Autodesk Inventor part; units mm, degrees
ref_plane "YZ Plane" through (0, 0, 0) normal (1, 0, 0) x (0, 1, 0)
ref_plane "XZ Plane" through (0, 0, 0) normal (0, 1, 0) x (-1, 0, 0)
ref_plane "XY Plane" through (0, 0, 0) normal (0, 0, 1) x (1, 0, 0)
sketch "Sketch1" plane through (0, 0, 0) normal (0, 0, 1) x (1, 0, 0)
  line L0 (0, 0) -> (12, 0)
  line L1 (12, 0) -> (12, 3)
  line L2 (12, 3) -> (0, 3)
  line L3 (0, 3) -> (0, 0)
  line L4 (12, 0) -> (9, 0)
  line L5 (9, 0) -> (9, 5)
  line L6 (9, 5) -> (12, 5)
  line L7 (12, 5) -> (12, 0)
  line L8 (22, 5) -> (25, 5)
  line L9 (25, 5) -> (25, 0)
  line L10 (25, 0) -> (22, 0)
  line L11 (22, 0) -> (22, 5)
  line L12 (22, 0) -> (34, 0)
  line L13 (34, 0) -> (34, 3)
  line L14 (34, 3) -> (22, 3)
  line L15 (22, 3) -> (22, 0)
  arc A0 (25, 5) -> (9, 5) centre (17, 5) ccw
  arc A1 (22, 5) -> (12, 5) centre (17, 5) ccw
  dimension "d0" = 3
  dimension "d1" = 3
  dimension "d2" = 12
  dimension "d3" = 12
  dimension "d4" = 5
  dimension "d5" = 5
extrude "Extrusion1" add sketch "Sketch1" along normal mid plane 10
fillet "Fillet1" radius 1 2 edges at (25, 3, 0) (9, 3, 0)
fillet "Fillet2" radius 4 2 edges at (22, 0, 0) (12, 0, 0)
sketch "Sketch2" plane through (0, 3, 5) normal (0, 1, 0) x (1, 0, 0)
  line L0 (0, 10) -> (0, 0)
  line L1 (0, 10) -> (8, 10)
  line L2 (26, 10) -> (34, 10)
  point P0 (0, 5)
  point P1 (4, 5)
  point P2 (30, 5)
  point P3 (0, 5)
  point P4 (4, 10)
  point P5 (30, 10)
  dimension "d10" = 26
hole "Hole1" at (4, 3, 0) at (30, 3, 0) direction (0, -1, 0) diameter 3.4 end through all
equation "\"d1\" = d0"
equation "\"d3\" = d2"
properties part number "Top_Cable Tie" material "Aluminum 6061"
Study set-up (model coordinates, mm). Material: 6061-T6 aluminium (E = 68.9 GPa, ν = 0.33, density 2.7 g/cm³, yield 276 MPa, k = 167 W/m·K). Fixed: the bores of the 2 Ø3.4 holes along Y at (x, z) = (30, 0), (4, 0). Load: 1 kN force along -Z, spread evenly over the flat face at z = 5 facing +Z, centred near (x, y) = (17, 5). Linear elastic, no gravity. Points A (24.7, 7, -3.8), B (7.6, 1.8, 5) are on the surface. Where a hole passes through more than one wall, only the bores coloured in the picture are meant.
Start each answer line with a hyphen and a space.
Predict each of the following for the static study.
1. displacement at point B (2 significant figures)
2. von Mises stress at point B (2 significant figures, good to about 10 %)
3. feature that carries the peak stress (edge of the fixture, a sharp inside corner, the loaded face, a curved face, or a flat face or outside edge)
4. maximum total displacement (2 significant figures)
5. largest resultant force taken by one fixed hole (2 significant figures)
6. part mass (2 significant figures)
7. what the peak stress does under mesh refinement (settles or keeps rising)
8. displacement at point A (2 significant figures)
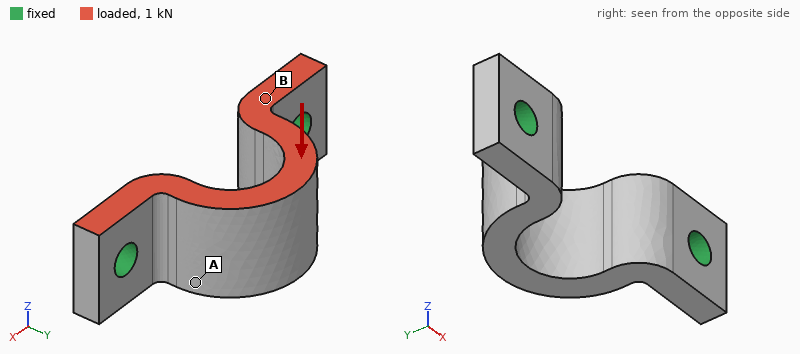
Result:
- 13 µm
- 88 MPa
- edge of the fixture
- 58 µm
- 500 N
- 3.6 g
- keeps rising
- 31 µm
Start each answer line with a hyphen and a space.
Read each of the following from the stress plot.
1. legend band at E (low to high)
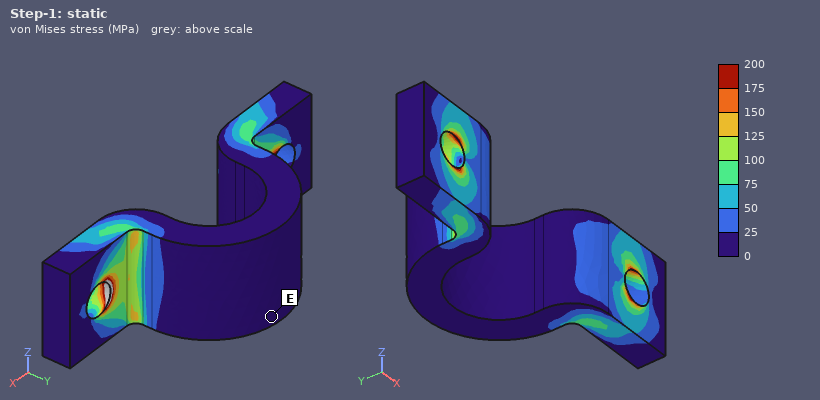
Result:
- 0 to 25 MPa
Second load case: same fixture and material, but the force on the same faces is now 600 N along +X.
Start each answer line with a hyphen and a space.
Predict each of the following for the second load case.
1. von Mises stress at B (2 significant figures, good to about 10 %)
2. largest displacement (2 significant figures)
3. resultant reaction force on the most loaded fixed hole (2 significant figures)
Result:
- 17 MPa
- 14 µm
- 320 N
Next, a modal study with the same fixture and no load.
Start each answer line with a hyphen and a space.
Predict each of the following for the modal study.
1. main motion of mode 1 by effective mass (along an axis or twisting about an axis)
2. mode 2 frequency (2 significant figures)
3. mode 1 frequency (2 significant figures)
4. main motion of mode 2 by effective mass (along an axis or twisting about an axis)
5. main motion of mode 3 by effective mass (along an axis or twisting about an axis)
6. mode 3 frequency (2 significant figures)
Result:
- along Z
- 26 kHz
- 13 kHz
- along X
- along Y
- 30 kHz
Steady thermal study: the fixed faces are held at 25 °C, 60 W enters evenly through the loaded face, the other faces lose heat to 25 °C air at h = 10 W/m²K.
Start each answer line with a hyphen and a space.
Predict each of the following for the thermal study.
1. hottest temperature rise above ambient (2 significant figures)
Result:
- 53 K
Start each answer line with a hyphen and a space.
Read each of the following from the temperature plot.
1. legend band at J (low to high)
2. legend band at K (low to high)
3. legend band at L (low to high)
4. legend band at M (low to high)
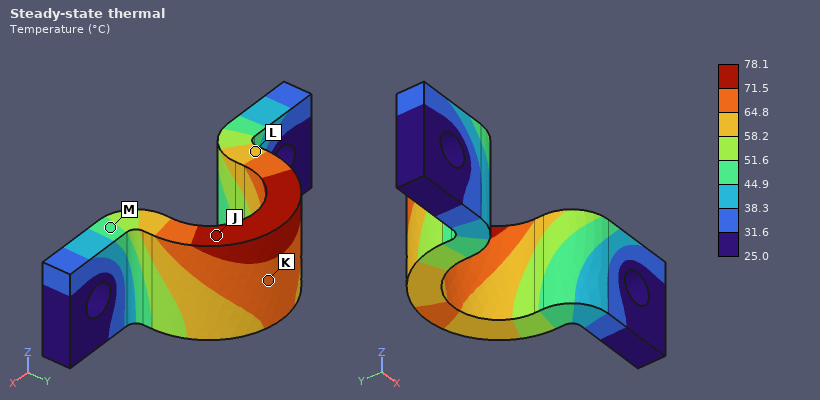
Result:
- 71.5 to 78.1 °C
- 64.8 to 71.5 °C
- 58.2 to 64.8 °C
- 44.9 to 51.6 °C
